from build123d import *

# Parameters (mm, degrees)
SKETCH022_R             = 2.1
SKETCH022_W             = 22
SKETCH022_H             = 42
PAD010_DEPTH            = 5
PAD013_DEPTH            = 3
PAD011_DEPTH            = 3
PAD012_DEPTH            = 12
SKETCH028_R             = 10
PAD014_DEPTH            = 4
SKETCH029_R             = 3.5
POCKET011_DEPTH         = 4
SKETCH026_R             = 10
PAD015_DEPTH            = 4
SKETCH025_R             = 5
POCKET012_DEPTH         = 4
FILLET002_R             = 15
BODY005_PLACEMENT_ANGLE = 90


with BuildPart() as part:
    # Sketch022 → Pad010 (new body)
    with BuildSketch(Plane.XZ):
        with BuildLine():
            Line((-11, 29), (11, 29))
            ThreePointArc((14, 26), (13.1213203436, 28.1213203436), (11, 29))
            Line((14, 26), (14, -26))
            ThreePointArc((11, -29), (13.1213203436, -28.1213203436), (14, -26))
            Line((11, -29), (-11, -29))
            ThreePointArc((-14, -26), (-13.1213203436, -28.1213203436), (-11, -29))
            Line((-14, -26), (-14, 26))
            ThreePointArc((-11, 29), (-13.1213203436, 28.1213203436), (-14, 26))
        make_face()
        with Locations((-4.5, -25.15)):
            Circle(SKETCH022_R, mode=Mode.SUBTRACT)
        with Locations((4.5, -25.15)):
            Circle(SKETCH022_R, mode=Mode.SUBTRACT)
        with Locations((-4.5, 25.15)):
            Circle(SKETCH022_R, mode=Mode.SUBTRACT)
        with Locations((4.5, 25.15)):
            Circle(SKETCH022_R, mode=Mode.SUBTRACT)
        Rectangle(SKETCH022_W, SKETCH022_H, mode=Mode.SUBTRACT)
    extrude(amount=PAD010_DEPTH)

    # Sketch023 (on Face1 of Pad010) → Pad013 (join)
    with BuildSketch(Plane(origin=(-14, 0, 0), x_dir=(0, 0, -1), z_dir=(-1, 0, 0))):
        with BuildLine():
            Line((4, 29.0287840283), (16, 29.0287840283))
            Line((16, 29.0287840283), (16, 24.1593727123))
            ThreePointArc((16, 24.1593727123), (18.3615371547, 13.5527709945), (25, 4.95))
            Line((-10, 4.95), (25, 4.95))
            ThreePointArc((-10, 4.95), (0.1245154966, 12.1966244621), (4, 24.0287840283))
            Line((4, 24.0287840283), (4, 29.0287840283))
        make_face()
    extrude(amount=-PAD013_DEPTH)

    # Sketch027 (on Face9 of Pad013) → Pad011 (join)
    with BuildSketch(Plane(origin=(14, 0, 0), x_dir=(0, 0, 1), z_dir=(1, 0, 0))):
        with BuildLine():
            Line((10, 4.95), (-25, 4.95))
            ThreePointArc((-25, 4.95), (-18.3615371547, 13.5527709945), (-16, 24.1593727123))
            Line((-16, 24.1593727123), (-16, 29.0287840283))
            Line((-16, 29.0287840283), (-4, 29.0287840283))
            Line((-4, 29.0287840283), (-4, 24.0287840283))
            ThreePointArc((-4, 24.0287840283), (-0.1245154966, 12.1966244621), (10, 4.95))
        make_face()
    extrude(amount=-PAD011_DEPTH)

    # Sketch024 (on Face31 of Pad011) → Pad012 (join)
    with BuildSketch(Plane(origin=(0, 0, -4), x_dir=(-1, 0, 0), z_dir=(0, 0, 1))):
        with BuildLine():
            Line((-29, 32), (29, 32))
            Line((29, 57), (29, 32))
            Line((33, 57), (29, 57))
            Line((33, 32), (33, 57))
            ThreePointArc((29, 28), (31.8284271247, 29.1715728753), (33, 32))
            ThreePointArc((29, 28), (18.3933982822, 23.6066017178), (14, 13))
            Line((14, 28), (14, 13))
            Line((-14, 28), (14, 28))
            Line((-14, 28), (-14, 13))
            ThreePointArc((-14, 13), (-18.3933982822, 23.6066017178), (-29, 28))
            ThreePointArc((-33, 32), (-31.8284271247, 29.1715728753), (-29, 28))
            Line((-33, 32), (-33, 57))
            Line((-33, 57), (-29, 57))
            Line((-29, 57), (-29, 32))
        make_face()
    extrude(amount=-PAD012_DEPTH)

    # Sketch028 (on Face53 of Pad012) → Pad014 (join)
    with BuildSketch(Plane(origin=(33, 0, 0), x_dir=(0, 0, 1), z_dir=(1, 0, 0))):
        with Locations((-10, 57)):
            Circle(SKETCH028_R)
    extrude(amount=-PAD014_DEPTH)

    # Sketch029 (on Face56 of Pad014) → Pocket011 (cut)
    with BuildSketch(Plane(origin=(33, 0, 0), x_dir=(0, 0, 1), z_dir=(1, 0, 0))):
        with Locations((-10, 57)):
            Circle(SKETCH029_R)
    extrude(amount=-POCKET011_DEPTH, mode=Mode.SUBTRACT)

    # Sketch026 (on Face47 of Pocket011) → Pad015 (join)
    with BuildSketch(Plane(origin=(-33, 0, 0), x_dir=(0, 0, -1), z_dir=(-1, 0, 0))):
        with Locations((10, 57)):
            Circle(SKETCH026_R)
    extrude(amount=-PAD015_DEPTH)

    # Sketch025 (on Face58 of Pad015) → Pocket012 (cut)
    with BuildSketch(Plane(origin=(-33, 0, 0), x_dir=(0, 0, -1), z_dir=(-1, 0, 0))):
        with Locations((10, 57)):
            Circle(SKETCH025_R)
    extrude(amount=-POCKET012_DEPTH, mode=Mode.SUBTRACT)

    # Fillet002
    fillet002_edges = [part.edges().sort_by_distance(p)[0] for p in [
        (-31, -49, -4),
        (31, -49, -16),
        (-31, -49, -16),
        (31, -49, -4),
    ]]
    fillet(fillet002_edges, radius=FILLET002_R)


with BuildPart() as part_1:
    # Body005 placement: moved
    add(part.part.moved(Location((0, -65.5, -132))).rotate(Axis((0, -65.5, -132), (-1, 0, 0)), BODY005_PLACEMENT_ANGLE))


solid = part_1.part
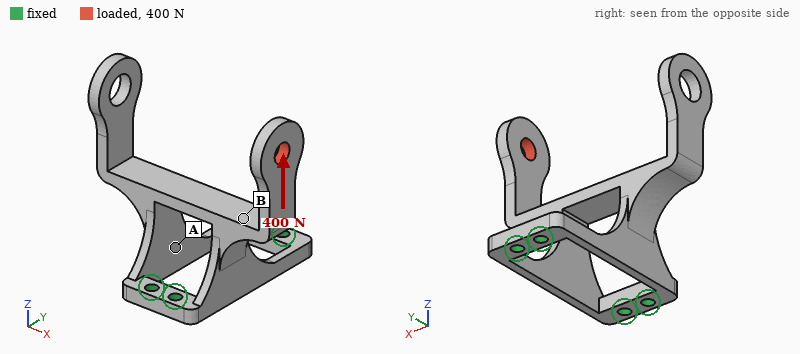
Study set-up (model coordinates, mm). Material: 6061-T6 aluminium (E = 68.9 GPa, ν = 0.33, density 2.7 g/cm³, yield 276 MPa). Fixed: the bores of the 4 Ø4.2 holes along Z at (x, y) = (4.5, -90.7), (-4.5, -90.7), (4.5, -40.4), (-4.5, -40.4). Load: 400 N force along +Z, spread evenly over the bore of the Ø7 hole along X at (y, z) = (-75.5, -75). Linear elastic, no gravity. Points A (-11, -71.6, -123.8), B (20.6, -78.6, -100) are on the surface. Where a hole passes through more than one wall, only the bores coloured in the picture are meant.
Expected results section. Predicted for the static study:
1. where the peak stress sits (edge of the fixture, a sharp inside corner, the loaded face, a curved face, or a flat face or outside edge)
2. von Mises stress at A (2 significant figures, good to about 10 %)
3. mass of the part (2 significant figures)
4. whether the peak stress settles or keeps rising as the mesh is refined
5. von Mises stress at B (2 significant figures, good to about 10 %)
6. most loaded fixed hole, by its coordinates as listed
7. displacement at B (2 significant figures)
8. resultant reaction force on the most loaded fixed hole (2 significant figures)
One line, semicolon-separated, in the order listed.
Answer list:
edge of the fixture; 15 MPa; 36 g; keeps rising; 54 MPa; (4.5, -90.7); 0.21 mm; 560 N
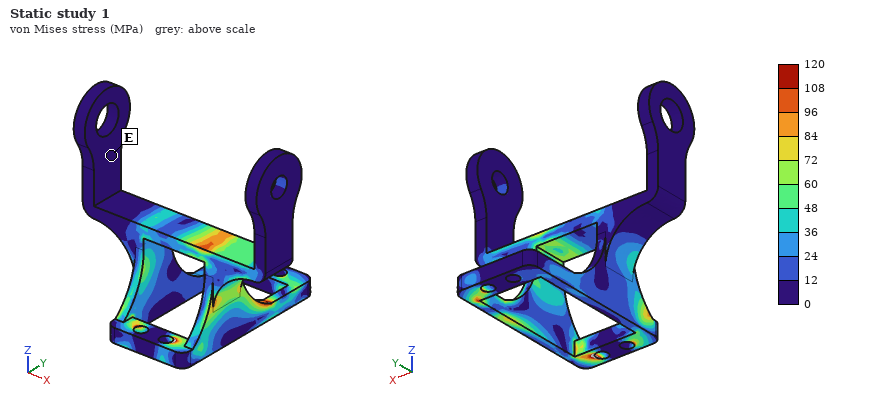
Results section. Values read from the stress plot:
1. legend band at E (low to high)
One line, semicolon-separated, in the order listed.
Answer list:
0 to 12 MPa
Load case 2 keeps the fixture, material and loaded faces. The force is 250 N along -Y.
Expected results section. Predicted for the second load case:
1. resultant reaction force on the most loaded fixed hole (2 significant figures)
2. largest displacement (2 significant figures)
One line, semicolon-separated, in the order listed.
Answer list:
390 N; 0.87 mm
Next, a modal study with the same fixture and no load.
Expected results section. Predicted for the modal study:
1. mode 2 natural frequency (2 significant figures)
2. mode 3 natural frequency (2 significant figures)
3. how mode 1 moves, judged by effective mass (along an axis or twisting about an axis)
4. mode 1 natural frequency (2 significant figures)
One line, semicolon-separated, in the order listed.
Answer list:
1400 Hz; 1500 Hz; along X; 910 Hz
